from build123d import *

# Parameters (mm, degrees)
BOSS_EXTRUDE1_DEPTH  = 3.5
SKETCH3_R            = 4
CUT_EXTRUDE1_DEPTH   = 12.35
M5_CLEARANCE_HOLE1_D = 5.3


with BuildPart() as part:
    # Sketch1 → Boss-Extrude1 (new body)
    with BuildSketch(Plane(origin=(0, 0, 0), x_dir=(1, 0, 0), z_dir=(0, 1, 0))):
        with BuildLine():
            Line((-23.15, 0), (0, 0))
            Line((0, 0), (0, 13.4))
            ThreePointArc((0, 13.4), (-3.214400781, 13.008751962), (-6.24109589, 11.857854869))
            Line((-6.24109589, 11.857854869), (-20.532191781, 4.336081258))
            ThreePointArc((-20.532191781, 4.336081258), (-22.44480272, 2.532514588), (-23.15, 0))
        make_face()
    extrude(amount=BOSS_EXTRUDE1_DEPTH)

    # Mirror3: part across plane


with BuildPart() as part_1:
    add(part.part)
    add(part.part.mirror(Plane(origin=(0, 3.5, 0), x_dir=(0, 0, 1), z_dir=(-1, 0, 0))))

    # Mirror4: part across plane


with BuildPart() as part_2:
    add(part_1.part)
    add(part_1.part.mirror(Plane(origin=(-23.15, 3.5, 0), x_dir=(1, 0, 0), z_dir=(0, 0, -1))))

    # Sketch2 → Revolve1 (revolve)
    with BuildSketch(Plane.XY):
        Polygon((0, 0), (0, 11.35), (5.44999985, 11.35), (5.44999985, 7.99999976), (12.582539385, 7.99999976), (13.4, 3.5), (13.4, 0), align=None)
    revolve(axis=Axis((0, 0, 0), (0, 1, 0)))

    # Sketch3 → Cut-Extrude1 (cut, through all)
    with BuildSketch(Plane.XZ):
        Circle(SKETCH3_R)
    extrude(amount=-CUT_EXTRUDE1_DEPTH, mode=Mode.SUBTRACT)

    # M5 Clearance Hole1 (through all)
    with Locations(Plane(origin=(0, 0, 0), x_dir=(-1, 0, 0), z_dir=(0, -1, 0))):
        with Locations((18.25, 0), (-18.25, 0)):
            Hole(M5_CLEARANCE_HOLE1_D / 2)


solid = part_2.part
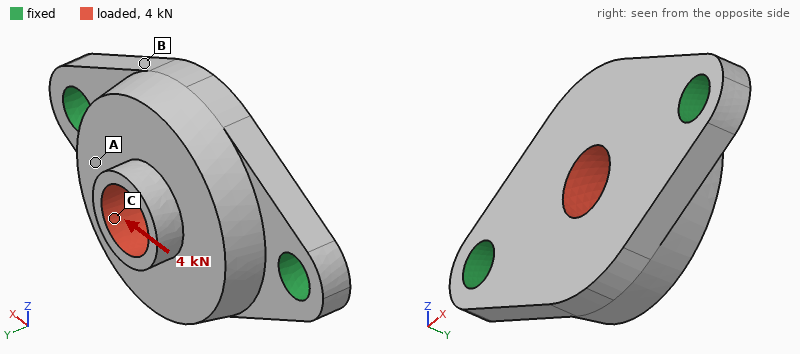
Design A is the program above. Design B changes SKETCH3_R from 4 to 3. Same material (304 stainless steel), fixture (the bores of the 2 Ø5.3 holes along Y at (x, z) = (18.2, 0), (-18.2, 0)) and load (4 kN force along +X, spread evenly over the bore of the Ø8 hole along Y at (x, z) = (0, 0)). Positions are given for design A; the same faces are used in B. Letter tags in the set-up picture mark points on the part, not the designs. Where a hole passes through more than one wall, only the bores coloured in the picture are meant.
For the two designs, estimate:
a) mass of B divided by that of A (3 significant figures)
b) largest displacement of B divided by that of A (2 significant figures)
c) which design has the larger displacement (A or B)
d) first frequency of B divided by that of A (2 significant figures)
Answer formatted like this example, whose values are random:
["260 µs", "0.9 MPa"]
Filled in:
["1.05", "0.82", "A", "0.99"]
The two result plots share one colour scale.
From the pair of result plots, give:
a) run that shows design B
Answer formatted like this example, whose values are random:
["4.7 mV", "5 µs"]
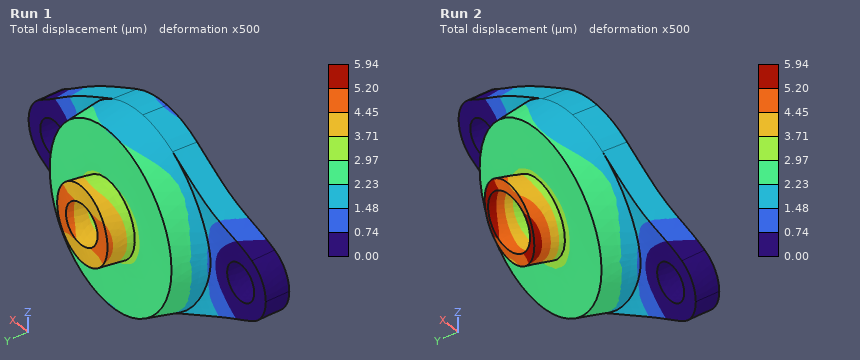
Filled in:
["Run 1"]
